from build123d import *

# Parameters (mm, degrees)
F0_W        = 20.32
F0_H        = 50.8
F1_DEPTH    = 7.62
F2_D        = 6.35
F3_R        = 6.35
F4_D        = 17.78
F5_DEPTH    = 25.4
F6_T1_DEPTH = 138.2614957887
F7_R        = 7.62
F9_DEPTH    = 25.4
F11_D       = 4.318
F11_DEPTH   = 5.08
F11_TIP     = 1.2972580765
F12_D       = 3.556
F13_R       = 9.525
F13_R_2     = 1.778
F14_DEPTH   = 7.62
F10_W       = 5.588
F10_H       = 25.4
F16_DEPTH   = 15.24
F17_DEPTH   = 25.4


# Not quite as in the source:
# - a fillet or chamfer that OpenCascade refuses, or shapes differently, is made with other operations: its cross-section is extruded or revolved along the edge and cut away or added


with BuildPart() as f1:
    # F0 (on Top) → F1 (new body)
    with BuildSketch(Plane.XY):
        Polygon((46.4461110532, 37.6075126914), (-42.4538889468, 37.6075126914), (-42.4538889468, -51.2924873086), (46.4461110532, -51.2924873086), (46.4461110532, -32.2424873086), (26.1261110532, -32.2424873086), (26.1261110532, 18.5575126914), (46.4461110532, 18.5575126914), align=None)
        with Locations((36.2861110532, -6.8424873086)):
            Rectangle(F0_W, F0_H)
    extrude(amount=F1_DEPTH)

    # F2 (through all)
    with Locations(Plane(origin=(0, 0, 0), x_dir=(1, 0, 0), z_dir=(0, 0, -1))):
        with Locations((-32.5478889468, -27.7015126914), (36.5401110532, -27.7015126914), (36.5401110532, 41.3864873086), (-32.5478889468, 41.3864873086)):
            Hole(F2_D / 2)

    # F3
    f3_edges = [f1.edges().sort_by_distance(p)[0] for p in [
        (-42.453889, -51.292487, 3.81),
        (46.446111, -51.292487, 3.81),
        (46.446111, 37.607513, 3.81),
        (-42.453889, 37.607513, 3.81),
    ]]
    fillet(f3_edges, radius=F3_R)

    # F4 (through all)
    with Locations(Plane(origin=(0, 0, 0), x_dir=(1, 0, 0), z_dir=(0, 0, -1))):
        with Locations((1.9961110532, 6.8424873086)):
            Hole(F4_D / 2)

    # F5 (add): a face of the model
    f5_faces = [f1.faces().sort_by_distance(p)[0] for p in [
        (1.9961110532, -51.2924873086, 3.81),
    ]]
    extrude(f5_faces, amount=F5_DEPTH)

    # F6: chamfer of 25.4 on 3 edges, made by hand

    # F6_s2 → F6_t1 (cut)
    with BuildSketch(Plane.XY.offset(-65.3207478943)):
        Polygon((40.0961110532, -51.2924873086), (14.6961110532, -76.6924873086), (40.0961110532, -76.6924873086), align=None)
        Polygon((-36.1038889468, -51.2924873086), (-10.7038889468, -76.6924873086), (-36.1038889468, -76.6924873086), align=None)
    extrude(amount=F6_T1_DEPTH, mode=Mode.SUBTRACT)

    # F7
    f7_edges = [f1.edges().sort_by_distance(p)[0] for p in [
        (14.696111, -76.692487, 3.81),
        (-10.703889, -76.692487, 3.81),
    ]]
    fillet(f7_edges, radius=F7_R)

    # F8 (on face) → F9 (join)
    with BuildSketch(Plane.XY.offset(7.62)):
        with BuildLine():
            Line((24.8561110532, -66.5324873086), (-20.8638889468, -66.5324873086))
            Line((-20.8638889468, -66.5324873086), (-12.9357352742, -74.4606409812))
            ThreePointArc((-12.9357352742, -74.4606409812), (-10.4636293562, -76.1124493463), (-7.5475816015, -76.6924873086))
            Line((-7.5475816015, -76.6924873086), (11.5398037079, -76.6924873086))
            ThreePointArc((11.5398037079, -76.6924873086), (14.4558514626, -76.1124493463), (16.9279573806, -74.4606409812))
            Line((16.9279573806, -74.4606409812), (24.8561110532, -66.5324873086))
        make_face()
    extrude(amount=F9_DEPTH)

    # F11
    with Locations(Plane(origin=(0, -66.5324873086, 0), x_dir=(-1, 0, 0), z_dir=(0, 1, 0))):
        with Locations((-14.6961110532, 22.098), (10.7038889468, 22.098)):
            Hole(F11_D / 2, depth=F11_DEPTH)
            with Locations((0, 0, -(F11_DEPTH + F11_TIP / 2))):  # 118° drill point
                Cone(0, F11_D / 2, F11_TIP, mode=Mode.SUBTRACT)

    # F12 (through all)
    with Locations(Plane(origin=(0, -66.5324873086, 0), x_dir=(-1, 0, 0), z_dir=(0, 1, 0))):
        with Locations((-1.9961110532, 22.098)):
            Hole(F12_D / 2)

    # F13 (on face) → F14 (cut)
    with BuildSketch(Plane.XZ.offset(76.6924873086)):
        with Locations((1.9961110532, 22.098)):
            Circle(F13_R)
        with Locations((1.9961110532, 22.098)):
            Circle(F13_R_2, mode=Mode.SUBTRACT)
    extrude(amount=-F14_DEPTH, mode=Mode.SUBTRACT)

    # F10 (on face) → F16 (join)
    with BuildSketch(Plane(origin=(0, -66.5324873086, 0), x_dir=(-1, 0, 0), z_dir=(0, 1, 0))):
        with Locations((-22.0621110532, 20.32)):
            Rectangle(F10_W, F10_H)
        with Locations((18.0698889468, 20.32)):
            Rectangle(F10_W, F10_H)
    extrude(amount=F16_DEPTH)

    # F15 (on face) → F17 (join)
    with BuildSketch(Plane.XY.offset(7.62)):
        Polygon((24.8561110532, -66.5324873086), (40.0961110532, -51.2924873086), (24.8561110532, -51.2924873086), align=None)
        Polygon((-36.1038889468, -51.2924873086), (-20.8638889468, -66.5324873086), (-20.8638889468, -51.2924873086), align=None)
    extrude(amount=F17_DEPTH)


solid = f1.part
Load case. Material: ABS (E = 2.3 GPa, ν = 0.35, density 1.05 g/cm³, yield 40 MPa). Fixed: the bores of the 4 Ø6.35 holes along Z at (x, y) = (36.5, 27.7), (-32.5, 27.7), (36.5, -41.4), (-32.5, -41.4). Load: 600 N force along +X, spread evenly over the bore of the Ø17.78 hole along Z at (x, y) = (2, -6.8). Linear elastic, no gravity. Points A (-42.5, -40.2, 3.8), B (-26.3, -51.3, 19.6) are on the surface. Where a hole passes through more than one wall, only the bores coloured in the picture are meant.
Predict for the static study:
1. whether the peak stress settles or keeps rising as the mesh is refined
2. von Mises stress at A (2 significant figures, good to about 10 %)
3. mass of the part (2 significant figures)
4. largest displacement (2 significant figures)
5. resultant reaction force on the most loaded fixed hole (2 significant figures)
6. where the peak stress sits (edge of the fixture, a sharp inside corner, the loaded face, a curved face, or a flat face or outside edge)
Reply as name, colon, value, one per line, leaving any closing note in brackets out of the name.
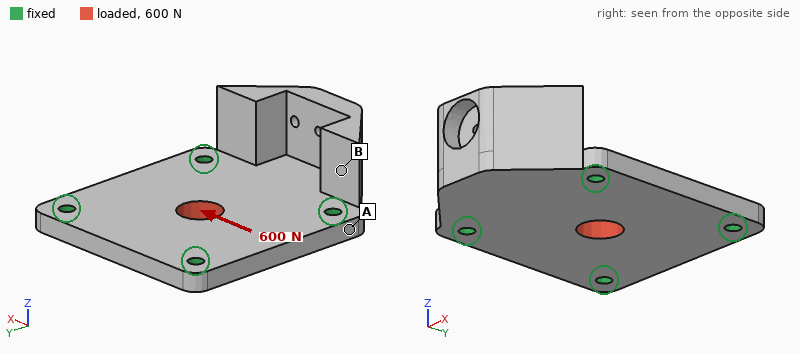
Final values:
whether the peak stress settles or keeps rising as the mesh is refined: keeps rising
von Mises stress at A: 0.88 MPa
mass of the part: 88 g
largest displacement: 26 µm
resultant reaction force on the most loaded fixed hole: 170 N
where the peak stress sits: edge of the fixture
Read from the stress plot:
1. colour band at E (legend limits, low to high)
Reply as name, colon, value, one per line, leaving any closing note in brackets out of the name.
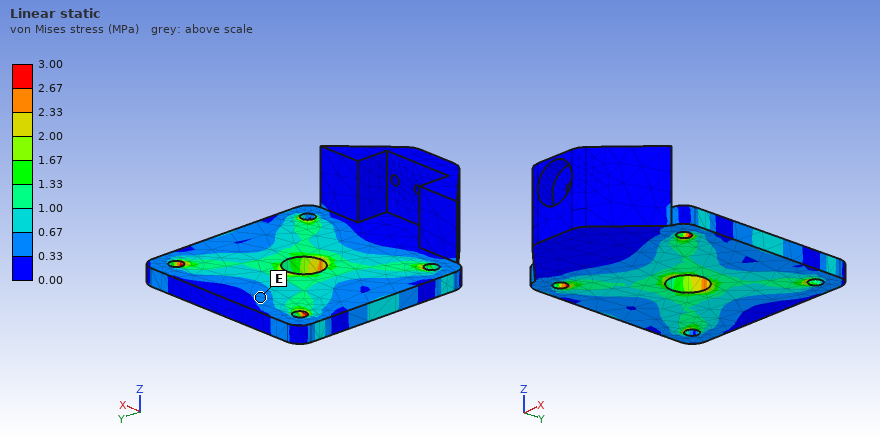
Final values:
colour band at E: 0.33 to 0.67 MPa
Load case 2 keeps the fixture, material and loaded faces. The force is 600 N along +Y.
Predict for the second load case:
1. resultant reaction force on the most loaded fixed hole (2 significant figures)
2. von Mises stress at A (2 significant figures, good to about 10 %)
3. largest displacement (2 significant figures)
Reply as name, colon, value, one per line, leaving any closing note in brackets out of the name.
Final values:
resultant reaction force on the most loaded fixed hole: 170 N
von Mises stress at A: 0.34 MPa
largest displacement: 25 µm
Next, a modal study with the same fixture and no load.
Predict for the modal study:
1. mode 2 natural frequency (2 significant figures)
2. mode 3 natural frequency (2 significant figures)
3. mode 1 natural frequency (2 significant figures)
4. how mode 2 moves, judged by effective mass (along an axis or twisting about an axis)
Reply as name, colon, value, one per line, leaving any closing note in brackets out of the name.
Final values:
mode 2 natural frequency: 1700 Hz
mode 3 natural frequency: 1900 Hz
mode 1 natural frequency: 750 Hz
how mode 2 moves, judged by effective mass: along Z
